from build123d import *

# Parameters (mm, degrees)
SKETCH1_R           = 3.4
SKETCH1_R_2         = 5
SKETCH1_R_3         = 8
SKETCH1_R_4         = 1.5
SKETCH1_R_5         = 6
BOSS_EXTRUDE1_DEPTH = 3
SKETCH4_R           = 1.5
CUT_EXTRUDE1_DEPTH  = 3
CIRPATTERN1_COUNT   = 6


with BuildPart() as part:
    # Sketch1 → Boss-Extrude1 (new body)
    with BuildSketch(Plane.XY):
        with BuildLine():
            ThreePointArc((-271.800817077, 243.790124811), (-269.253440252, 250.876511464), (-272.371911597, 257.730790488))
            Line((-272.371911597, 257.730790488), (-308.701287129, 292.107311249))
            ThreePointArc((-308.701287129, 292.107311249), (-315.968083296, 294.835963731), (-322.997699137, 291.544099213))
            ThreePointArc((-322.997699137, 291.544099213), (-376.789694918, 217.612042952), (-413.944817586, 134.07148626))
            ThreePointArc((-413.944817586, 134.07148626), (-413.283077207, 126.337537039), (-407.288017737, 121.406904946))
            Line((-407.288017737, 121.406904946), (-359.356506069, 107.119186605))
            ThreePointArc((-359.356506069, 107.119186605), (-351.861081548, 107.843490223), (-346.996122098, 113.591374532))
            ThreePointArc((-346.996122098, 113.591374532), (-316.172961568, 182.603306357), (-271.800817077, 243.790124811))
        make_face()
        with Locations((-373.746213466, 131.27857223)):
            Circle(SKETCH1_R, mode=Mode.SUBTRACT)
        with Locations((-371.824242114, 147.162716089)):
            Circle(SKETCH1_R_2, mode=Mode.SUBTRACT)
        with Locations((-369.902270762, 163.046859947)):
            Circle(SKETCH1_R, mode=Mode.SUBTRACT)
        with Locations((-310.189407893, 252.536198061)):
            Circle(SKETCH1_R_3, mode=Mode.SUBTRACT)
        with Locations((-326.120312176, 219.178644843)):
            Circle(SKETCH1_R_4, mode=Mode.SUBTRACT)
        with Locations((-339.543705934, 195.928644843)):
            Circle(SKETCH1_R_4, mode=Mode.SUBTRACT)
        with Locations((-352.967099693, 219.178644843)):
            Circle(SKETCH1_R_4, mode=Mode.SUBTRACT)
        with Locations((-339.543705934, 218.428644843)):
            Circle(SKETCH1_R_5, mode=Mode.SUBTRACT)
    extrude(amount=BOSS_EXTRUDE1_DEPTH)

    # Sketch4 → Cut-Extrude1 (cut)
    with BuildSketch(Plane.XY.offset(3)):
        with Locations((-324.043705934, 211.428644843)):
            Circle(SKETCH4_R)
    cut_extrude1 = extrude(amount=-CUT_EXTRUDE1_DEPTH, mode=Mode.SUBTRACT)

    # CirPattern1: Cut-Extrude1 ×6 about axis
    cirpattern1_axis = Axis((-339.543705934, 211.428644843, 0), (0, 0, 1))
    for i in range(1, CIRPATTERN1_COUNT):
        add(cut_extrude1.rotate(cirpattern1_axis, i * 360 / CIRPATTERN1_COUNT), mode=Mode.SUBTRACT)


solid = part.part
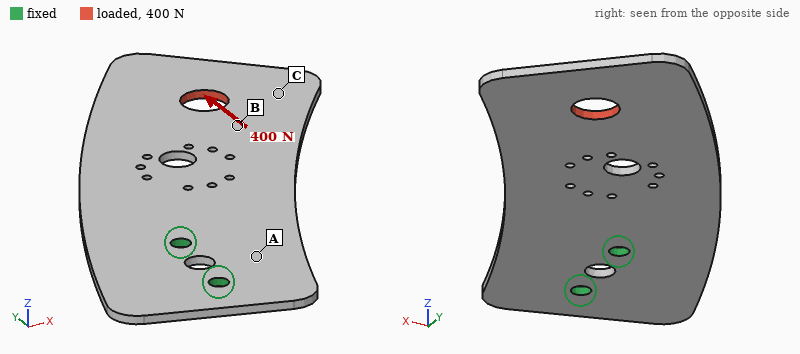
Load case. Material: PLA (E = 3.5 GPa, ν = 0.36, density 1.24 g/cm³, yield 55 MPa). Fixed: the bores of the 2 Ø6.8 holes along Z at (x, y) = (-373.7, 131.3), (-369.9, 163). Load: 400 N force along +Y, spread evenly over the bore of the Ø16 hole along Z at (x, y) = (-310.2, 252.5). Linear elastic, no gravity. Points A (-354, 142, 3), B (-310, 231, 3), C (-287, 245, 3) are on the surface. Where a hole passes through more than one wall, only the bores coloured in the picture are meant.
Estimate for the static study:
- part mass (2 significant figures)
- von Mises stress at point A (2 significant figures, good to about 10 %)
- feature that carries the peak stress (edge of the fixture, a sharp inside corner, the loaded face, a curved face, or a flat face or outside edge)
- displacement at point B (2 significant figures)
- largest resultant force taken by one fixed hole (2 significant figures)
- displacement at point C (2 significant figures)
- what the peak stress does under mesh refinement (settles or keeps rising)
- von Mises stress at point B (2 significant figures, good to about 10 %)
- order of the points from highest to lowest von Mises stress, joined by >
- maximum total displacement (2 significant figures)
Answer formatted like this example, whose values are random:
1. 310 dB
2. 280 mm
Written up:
1. 46 g
2. 9.2 MPa
3. edge of the fixture
4. 0.73 mm
5. 700 N
6. 0.98 mm
7. keeps rising
8. 3.9 MPa
9. A > B > C
10. 1.2 mm
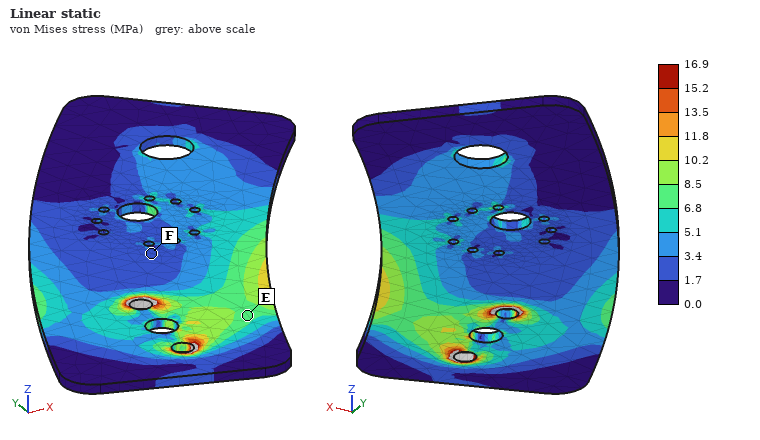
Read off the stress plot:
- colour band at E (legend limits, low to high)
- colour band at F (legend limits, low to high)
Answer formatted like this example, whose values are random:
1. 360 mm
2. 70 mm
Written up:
1. 6.8 to 8.5 MPa
2. 1.7 to 3.4 MPa
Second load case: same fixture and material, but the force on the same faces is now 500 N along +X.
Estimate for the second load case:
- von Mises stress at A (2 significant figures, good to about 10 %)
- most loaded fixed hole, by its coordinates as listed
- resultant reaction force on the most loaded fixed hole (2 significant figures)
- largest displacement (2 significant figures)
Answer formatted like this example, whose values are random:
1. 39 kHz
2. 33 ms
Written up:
1. 15 MPa
2. (-369.9, 163)
3. 1.7 kN
4. 2.4 mm
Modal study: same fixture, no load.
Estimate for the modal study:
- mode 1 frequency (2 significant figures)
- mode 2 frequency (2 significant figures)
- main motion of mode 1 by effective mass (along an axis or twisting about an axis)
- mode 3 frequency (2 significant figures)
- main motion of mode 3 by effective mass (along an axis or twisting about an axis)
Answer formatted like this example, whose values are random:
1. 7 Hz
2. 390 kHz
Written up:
1. 44 Hz
2. 160 Hz
3. along Z
4. 260 Hz
5. along Z
